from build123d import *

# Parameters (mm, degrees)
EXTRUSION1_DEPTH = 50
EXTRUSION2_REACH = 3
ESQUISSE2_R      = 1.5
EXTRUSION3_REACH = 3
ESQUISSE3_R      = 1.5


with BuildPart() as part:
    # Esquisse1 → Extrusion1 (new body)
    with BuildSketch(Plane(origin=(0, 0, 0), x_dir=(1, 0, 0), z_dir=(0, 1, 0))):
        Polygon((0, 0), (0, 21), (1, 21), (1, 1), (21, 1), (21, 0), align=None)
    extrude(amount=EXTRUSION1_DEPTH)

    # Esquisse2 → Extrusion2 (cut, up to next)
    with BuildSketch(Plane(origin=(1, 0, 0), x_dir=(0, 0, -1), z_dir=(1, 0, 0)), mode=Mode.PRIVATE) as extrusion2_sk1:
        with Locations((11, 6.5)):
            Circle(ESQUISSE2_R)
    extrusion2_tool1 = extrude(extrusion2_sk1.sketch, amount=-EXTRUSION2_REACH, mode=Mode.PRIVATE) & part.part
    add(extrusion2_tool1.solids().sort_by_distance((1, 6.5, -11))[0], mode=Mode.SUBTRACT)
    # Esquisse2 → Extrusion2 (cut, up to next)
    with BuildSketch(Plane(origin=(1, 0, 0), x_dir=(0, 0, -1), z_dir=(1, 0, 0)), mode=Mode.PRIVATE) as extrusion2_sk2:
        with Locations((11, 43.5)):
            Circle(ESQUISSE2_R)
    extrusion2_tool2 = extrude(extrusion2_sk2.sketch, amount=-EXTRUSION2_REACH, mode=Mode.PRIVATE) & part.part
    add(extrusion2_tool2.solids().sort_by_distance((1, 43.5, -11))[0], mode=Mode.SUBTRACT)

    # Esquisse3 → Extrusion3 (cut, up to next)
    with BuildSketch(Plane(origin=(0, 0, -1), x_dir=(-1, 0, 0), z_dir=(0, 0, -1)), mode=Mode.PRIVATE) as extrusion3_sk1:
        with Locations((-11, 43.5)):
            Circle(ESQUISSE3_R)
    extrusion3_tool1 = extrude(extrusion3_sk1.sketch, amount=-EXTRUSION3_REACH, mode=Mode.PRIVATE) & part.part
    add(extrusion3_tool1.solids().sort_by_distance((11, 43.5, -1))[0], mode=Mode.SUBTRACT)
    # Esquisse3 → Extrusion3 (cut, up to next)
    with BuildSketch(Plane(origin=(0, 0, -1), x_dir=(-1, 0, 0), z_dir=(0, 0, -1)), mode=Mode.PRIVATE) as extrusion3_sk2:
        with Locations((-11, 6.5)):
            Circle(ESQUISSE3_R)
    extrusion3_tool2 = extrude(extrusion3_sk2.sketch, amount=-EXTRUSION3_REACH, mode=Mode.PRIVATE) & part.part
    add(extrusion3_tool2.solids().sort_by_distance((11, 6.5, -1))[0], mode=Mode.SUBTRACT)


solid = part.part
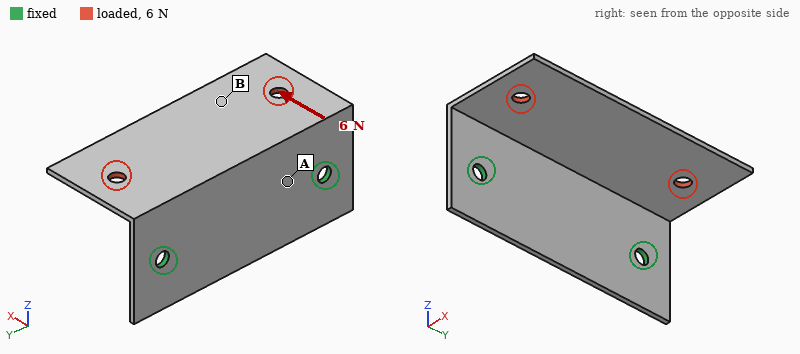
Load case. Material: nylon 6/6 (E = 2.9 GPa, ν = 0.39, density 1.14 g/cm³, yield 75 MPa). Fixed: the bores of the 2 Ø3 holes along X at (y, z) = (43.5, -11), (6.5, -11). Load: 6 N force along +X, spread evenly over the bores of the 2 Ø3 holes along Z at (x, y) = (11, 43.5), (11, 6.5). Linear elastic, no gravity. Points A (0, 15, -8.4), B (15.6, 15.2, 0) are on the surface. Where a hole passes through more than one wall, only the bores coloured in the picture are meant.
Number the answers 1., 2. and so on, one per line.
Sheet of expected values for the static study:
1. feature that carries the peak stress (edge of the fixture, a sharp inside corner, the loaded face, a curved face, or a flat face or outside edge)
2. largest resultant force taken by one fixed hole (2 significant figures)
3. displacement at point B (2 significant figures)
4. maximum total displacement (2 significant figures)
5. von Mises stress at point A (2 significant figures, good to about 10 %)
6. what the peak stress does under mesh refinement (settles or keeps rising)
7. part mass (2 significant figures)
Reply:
1. edge of the fixture
2. 3.0 N
3. 0.48 mm
4. 0.65 mm
5. 2.8 MPa
6. keeps rising
7. 2.3 g
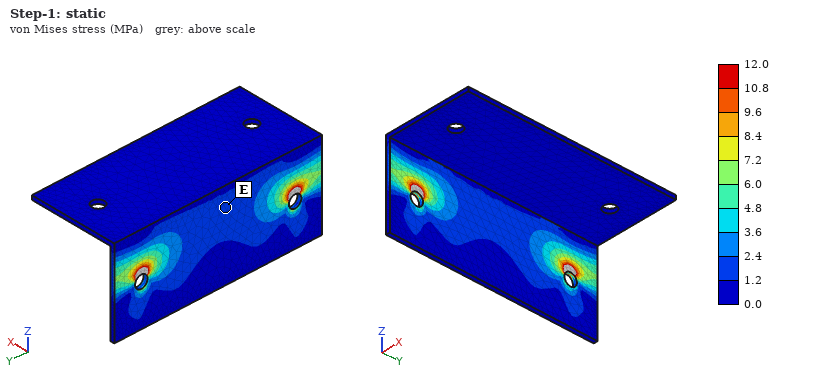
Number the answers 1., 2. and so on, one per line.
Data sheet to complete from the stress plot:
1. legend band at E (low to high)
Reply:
1. 1.2 to 2.4 MPa
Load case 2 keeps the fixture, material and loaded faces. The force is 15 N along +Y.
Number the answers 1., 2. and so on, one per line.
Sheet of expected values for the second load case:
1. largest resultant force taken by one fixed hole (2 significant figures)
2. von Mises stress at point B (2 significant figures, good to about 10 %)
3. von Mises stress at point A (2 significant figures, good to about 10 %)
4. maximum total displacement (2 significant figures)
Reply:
1. 9.5 N
2. 1.2 MPa
3. 2.1 MPa
4. 0.57 mm
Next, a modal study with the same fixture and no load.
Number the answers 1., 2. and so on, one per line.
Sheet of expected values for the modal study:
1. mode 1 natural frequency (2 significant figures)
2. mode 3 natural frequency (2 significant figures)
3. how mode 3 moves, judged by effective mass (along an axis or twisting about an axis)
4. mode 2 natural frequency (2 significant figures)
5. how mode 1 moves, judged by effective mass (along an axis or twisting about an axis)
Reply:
1. 340 Hz
2. 1000 Hz
3. along X
4. 590 Hz
5. along Z
